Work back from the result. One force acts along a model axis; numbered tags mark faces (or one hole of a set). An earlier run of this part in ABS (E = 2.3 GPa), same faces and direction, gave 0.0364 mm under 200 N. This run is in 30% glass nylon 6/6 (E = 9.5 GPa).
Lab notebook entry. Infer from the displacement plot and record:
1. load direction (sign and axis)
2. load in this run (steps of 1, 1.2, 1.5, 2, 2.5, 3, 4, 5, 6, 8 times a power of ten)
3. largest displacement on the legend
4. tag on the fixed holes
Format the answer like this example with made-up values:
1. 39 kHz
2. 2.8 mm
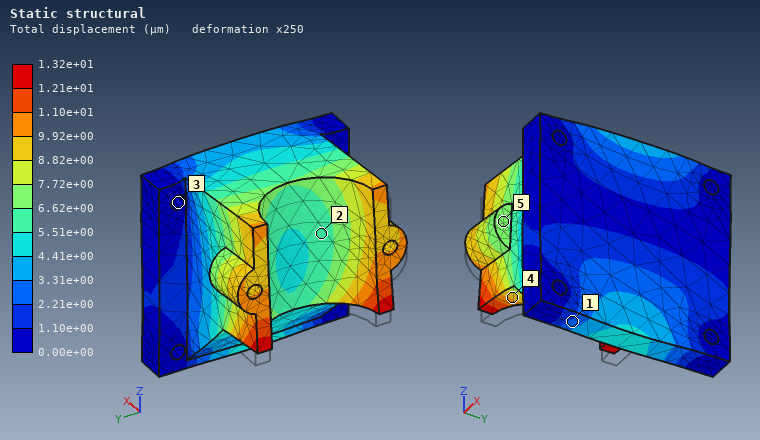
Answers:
1. +Z
2. 300 N
3. 1.32e+01 µm
4. 3
